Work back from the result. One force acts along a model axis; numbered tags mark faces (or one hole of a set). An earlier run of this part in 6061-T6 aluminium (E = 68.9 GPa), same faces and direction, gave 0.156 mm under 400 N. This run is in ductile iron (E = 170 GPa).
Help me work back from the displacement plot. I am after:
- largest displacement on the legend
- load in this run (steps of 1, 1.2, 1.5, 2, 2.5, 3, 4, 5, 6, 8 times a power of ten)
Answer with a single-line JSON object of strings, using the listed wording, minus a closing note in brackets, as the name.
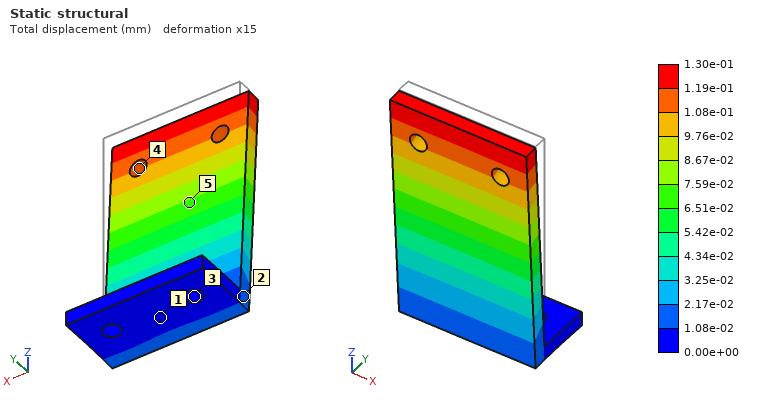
{"largest displacement on the legend": "1.30e-01 mm", "load in this run": "800 N"}
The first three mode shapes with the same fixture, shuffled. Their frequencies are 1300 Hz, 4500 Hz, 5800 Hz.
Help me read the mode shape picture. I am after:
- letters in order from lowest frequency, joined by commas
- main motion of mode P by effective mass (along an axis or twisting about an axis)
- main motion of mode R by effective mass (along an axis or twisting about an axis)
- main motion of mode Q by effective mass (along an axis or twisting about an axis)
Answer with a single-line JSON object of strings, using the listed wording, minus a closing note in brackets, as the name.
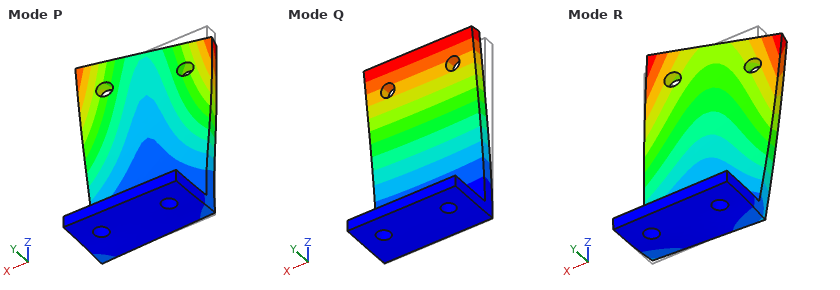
{"letters in order from lowest frequency, joined by commas": "Q, R, P", "main motion of mode P by effective mass": "along X", "main motion of mode R by effective mass": "along X", "main motion of mode Q by effective mass": "along Y"}
